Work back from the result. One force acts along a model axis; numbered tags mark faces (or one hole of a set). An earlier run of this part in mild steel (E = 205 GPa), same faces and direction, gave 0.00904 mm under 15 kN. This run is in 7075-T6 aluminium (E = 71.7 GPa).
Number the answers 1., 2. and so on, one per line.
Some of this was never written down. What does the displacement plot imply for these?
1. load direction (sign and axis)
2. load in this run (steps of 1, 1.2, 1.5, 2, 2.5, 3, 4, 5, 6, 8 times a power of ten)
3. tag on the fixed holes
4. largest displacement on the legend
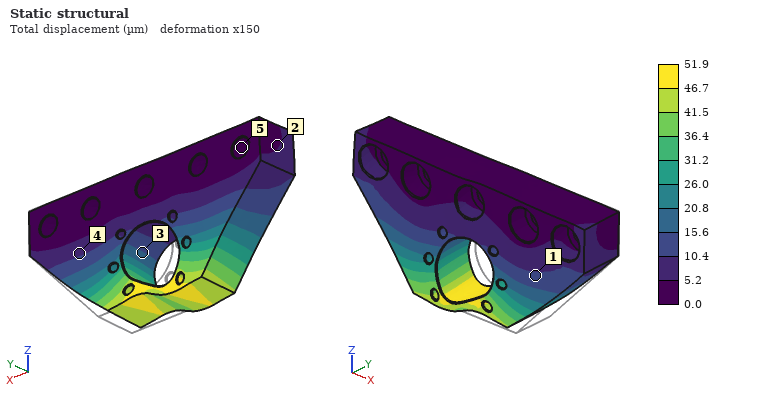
1. -X
2. 30 kN
3. 5
4. 51.9 µm
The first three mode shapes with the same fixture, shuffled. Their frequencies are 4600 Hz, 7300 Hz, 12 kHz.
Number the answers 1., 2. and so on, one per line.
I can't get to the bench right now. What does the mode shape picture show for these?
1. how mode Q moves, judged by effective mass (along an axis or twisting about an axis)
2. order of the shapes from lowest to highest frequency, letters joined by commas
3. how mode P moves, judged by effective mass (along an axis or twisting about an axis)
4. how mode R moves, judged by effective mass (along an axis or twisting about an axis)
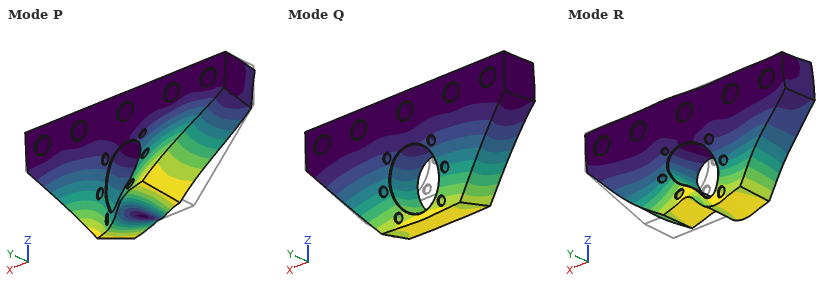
1. along Y
2. Q, P, R
3. twisting about Z
4. along X
